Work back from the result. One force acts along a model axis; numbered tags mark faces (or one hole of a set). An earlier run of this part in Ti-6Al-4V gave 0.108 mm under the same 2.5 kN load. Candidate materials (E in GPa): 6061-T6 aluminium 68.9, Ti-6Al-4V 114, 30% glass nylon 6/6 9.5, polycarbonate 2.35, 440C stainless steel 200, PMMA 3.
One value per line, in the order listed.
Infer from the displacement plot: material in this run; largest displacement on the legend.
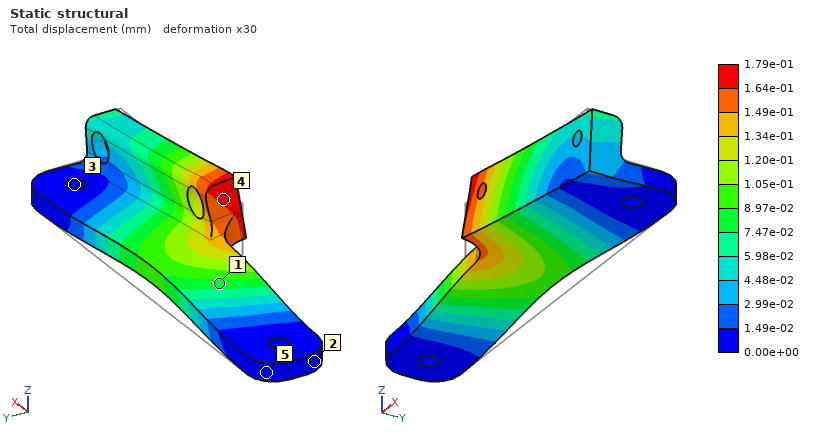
6061-T6 aluminium
1.79e-01 mm
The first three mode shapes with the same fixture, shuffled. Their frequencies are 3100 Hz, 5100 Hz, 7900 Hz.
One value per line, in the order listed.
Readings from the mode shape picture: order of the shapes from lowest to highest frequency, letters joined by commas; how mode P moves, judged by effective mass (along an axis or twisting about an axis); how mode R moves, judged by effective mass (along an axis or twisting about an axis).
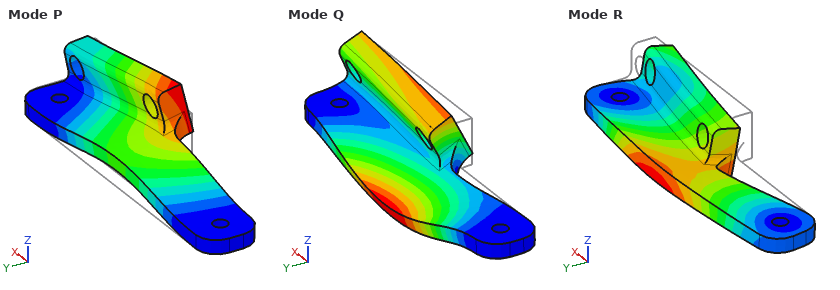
P, Q, R
along Z
along Y
